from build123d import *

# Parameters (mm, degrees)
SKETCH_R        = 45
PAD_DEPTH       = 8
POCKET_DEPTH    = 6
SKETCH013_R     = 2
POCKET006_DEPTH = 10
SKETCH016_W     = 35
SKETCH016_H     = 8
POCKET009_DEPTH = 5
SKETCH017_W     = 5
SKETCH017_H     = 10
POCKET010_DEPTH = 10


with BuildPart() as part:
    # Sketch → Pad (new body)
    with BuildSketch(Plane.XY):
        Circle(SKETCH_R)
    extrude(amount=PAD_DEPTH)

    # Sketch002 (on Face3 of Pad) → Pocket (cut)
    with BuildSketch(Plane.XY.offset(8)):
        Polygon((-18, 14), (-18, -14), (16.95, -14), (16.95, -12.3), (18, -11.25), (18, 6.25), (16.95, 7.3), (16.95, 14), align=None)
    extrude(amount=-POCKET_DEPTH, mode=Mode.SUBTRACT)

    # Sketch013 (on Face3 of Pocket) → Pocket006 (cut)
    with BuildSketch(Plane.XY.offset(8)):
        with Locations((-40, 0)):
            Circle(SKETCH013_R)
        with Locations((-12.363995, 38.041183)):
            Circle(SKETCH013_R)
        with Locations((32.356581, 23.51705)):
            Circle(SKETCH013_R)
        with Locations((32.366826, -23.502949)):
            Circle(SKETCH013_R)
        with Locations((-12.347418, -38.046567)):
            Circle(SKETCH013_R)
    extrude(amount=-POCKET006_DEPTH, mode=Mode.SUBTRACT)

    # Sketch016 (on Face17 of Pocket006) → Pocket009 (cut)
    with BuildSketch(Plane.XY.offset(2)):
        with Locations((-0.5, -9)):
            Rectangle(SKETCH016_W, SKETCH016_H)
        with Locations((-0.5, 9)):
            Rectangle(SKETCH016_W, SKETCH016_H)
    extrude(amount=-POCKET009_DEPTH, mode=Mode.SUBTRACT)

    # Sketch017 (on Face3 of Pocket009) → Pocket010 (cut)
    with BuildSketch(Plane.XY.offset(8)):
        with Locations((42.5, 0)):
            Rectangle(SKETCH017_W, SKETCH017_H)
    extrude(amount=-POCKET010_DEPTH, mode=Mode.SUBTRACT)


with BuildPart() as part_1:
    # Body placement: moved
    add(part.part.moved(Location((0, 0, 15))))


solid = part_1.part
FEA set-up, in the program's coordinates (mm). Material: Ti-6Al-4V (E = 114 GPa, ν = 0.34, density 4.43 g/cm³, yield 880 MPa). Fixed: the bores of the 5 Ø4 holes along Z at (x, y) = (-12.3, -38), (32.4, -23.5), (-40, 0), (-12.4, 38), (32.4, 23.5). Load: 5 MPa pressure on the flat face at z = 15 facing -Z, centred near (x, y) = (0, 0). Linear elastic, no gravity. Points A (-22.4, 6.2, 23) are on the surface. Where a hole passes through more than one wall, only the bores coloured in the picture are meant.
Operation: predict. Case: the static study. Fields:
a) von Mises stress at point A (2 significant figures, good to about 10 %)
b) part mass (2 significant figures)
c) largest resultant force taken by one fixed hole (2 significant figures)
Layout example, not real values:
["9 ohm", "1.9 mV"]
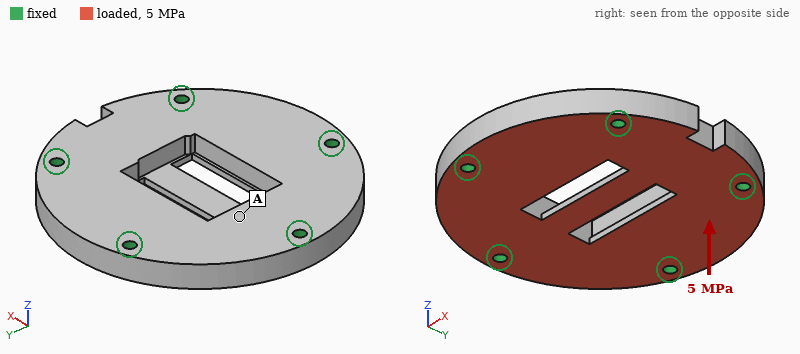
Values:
["66 MPa", "190 g", "6.0 kN"]
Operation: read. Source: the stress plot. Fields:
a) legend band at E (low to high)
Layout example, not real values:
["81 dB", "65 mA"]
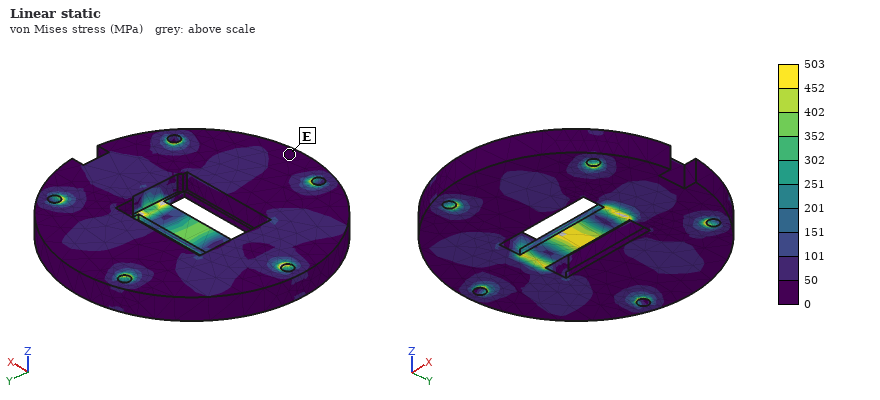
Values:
["0 to 50 MPa"]
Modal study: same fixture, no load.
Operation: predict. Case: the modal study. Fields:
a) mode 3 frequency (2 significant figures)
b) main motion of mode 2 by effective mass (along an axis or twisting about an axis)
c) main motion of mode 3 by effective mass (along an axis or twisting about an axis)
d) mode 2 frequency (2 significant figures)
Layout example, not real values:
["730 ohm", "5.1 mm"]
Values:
["13 kHz", "along Z", "twisting about X", "11 kHz"]
